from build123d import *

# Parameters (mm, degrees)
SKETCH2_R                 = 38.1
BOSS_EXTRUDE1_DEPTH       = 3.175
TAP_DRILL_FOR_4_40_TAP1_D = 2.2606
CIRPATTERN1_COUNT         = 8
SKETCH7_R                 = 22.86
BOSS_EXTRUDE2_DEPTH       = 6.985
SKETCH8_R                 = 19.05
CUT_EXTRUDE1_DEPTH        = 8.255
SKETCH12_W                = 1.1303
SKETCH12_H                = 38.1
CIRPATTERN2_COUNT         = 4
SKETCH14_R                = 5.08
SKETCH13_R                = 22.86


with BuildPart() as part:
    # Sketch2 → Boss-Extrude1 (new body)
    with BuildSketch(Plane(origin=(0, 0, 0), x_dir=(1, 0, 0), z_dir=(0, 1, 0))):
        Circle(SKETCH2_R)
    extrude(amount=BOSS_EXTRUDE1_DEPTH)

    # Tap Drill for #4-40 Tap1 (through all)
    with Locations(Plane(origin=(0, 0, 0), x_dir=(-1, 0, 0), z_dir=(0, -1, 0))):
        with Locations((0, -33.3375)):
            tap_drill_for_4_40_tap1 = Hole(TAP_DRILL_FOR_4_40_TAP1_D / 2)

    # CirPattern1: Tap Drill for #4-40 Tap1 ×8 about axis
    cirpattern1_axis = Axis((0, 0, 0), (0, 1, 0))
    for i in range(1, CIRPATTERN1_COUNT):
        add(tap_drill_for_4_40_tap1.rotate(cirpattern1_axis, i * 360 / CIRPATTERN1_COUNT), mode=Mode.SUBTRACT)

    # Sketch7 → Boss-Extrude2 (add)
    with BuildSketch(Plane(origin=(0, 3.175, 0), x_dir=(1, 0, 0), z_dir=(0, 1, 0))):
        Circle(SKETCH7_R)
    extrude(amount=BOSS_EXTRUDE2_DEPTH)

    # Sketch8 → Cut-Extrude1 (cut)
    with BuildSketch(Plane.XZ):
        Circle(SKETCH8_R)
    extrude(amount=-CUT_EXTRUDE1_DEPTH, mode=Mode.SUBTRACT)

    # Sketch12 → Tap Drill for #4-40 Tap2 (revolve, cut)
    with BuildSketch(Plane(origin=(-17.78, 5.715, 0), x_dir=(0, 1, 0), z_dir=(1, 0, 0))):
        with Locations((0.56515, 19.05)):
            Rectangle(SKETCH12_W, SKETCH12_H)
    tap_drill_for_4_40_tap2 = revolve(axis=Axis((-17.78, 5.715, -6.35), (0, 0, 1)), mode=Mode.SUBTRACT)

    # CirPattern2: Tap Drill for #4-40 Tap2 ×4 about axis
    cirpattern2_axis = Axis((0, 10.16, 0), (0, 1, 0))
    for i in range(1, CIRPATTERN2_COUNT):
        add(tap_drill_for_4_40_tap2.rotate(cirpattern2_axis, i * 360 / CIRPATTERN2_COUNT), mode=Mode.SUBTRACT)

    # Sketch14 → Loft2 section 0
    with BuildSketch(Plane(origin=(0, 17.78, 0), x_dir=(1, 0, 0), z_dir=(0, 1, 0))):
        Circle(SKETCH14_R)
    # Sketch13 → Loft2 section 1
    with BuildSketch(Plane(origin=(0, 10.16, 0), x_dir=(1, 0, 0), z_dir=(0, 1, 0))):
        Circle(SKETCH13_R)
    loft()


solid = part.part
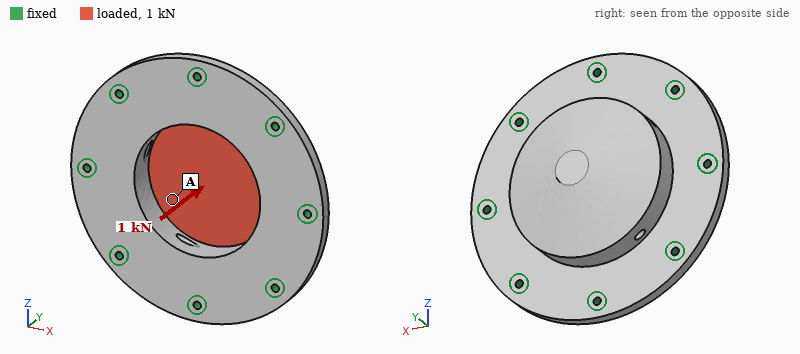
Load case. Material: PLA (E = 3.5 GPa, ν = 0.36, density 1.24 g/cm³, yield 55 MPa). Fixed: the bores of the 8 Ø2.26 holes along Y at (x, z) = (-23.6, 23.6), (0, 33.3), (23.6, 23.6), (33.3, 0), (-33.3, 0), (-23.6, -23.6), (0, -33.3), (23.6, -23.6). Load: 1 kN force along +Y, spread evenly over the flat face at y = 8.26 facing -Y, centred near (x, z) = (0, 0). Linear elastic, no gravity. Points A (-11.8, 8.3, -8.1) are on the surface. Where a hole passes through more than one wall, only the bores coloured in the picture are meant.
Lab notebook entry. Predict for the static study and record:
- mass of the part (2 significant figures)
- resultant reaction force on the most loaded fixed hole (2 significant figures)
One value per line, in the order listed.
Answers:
27 g
170 N
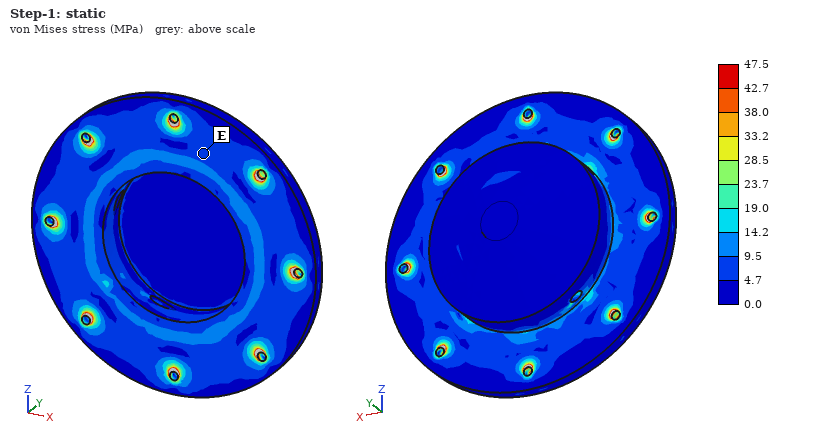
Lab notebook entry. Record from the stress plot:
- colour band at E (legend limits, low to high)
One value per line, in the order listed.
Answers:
4.7 to 9.5 MPa
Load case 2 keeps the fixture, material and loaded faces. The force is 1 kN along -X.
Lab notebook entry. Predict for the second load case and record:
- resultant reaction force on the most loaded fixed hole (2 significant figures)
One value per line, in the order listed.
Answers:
170 N
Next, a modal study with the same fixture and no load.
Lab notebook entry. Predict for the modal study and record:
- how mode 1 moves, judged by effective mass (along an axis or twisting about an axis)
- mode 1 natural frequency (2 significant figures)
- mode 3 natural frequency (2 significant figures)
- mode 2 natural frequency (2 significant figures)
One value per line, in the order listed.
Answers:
along Y
2700 Hz
3700 Hz
3700 Hz
